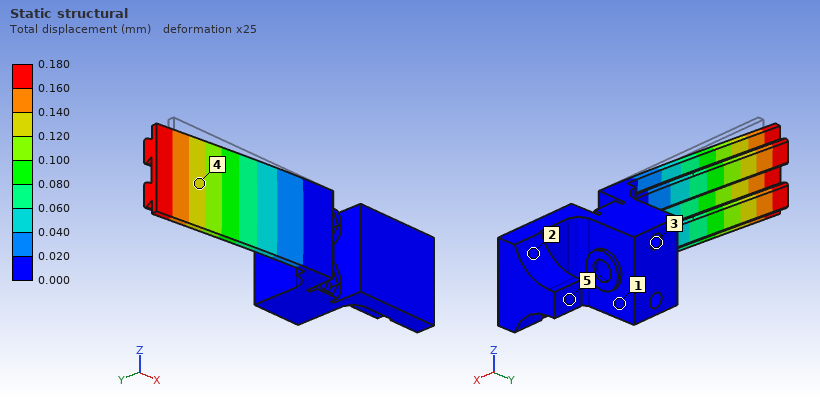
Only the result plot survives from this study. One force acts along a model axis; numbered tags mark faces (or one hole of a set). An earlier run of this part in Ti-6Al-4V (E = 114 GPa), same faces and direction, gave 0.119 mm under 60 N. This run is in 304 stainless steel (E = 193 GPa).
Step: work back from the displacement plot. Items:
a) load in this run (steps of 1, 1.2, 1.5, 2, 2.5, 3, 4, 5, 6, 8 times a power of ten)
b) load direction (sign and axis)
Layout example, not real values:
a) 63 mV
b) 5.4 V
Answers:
a) 150 N
b) +Y
